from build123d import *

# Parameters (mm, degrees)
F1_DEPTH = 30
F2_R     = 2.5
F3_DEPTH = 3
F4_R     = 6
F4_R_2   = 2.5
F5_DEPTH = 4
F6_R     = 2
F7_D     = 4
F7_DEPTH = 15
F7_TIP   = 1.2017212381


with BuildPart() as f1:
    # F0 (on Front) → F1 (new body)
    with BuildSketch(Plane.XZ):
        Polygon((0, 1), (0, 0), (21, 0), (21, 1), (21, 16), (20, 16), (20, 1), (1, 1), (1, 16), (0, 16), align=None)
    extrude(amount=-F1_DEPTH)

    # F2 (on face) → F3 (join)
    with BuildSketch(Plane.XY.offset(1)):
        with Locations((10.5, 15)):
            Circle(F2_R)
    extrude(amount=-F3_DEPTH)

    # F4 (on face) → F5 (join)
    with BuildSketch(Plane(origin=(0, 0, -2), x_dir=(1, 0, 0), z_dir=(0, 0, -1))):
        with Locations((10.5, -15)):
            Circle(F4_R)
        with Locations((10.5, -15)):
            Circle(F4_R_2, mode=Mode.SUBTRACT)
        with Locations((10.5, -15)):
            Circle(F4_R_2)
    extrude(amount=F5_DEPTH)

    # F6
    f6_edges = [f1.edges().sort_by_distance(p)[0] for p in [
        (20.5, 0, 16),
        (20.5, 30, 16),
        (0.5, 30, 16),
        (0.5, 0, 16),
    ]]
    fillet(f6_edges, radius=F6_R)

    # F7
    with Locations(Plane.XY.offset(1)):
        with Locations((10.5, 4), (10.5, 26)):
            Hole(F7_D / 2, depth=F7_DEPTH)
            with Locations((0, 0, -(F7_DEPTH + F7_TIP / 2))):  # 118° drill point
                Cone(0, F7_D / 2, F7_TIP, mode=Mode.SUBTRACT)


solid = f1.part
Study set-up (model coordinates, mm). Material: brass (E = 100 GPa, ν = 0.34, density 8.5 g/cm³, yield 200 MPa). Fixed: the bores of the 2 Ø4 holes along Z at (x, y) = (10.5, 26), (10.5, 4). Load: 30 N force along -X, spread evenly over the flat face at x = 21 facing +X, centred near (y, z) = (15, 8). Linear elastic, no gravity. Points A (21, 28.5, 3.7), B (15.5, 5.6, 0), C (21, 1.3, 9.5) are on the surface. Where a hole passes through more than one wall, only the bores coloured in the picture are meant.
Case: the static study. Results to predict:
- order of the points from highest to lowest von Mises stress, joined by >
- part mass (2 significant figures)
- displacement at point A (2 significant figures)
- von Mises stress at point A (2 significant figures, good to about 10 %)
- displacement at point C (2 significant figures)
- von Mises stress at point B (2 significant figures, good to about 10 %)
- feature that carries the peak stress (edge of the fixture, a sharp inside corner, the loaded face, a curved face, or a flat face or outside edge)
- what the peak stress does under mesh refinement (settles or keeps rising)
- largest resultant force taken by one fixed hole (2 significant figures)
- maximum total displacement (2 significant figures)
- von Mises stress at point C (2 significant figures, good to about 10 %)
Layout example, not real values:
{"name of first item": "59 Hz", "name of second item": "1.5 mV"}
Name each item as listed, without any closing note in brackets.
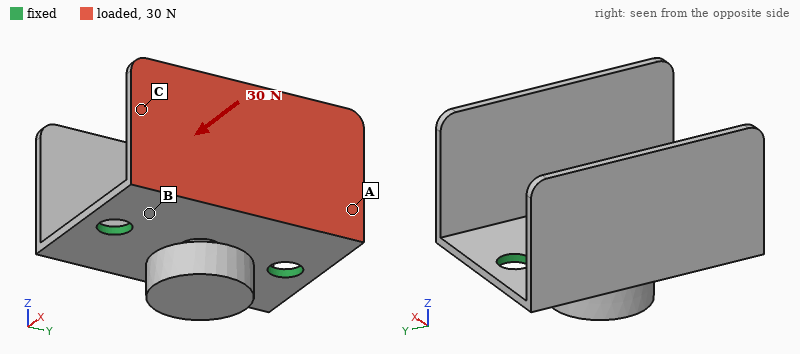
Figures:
{"order of the points from highest to lowest von Mises stress, joined by >": "B > A > C", "part mass": "17 g", "displacement at point A": "0.046 mm", "von Mises stress at point A": "25 MPa", "displacement at point C": "0.093 mm", "von Mises stress at point B": "40 MPa", "feature that carries the peak stress": "edge of the fixture", "what the peak stress does under mesh refinement": "keeps rising", "largest resultant force taken by one fixed hole": "16 N", "maximum total displacement": "0.16 mm", "von Mises stress at point C": "8.0 MPa"}
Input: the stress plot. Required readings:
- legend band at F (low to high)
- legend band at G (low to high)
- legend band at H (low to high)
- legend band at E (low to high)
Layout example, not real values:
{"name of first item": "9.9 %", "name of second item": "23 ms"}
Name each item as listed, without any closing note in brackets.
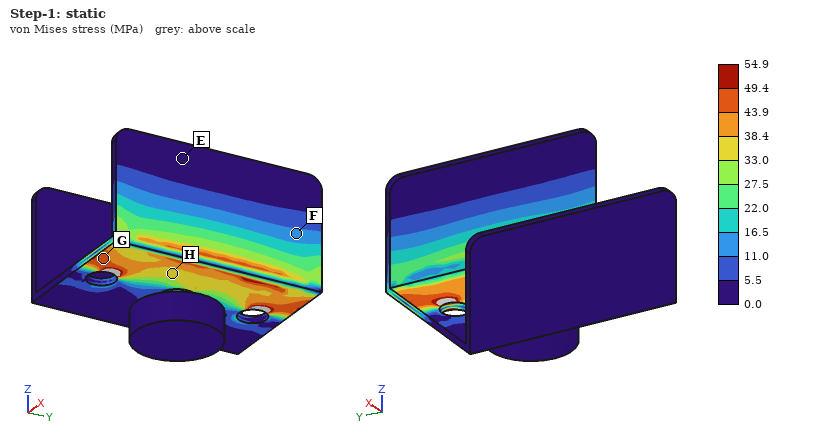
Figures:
{"legend band at F": "11.0 to 16.5 MPa", "legend band at G": "43.9 to 49.4 MPa", "legend band at H": "33.0 to 38.4 MPa", "legend band at E": "0.0 to 5.5 MPa"}
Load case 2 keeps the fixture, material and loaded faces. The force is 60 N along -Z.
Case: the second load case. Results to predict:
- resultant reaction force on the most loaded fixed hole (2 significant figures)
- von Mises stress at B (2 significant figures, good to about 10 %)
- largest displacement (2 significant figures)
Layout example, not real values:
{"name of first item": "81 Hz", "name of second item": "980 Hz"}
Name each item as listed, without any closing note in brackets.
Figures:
{"resultant reaction force on the most loaded fixed hole": "30 N", "von Mises stress at B": "67 MPa", "largest displacement": "0.18 mm"}
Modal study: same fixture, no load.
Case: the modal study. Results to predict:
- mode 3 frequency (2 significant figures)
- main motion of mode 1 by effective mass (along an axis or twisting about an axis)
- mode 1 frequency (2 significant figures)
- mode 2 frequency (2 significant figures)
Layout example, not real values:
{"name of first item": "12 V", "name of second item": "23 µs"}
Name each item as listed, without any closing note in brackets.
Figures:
{"mode 3 frequency": "2400 Hz", "main motion of mode 1 by effective mass": "along X", "mode 1 frequency": "1200 Hz", "mode 2 frequency": "1300 Hz"}
